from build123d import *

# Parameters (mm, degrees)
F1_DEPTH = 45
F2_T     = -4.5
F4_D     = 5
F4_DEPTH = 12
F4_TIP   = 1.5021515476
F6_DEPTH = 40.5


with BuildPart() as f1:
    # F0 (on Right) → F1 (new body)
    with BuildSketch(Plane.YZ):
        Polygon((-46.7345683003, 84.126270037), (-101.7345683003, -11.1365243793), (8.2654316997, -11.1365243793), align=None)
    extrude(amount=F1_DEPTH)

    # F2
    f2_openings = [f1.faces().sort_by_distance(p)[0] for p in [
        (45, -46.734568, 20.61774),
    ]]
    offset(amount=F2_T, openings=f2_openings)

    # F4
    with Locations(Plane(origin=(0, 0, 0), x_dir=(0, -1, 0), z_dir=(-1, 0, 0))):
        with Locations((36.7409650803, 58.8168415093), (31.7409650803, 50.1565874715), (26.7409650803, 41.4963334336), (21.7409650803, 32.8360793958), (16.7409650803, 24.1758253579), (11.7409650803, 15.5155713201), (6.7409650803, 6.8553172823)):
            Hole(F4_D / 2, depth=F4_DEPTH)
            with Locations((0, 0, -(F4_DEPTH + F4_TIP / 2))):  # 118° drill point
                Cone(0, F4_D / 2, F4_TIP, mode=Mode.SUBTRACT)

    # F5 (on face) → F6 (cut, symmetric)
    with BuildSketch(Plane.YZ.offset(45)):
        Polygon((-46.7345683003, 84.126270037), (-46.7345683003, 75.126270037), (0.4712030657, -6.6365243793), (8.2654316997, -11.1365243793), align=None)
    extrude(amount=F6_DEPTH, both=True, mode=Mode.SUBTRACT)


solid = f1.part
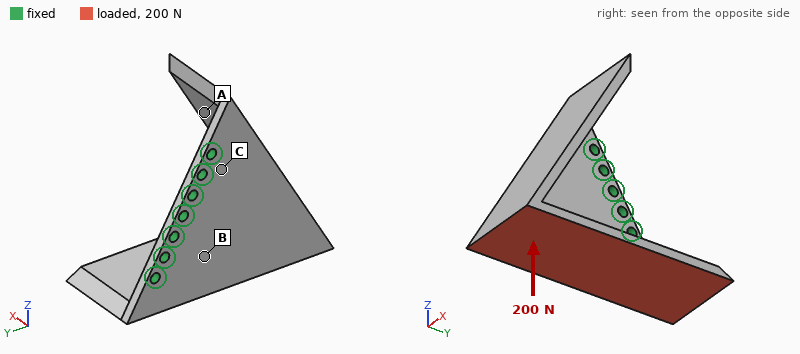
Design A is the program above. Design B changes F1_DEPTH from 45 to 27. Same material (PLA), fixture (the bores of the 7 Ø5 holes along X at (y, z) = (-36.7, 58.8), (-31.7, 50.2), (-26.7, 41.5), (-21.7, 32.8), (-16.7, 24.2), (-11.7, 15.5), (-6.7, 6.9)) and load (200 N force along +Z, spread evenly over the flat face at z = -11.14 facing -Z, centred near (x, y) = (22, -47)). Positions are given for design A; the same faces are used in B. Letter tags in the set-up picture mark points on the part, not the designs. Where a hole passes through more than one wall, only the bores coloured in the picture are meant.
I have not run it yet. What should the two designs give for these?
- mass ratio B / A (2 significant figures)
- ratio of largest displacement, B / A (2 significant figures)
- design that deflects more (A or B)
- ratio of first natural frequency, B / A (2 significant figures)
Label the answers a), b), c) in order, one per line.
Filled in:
a) 0.73
b) 0.33
c) A
d) 1.3
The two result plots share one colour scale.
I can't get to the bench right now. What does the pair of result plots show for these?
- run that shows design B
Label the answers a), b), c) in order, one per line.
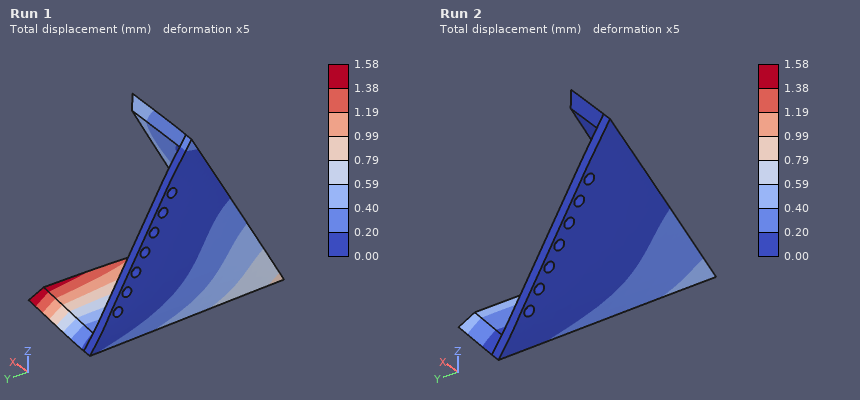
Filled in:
a) Run 2
